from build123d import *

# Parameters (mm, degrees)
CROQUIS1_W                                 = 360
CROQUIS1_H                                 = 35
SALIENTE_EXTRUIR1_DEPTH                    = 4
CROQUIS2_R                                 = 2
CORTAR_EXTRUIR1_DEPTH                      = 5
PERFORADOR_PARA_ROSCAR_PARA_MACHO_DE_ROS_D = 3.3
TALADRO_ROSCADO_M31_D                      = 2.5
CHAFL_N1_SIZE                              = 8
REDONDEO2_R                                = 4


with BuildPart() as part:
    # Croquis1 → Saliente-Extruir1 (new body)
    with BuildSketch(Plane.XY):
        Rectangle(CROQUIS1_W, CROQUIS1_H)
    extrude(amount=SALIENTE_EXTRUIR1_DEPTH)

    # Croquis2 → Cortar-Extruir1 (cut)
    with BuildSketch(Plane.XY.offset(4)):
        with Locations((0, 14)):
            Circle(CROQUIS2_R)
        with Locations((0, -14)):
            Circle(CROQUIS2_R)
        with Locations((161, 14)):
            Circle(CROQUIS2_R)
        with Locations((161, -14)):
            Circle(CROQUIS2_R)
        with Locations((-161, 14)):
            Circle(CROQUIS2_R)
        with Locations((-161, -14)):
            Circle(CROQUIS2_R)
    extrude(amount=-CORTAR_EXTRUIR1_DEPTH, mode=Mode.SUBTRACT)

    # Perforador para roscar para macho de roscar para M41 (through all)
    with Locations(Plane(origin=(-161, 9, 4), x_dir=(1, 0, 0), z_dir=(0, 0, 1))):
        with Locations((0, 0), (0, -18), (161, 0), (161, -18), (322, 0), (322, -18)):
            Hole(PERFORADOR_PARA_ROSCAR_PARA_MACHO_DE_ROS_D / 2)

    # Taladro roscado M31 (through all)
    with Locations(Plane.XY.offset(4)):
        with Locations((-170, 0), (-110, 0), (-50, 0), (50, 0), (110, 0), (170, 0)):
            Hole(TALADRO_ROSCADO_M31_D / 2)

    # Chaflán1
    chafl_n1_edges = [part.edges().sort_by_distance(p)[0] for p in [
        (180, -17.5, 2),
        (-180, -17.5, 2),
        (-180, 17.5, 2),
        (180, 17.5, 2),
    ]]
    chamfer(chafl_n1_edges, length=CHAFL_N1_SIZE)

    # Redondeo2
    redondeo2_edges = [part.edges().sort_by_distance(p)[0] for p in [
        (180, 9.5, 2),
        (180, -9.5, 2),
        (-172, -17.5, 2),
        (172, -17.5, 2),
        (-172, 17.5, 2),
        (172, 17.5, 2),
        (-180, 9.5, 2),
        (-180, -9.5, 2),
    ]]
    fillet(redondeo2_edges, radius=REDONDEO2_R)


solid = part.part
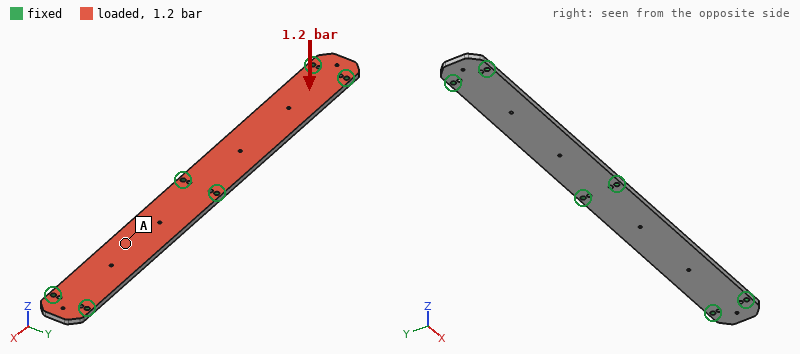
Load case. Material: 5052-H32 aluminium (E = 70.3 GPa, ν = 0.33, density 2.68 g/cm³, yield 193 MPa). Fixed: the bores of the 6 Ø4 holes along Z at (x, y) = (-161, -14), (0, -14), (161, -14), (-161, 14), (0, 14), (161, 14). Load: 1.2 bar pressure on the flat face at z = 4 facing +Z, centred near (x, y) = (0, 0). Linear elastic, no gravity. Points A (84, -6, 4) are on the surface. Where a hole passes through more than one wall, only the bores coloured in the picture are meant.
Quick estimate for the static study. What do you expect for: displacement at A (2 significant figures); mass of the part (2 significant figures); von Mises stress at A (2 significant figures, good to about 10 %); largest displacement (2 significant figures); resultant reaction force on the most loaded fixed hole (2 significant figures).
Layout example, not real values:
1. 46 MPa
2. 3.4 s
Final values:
1. 0.56 mm
2. 130 g
3. 47 MPa
4. 0.57 mm
5. 340 N
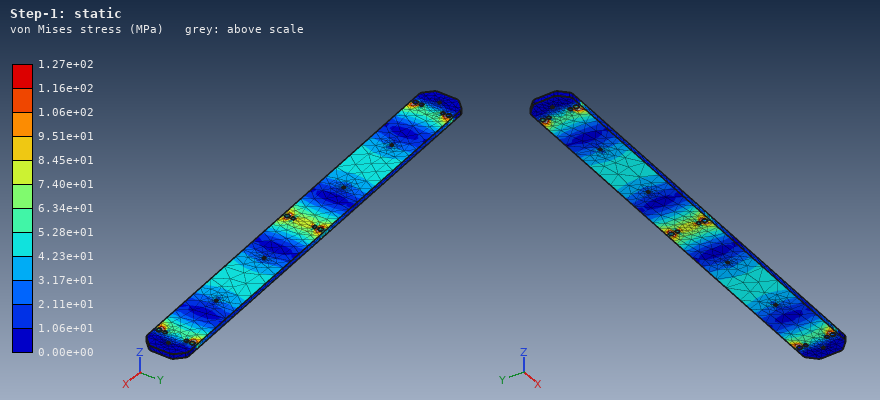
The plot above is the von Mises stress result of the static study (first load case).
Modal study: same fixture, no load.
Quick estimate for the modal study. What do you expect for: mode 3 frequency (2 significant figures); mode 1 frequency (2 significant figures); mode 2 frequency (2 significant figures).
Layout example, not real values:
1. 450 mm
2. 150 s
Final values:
1. 2200 Hz
2. 780 Hz
3. 810 Hz
